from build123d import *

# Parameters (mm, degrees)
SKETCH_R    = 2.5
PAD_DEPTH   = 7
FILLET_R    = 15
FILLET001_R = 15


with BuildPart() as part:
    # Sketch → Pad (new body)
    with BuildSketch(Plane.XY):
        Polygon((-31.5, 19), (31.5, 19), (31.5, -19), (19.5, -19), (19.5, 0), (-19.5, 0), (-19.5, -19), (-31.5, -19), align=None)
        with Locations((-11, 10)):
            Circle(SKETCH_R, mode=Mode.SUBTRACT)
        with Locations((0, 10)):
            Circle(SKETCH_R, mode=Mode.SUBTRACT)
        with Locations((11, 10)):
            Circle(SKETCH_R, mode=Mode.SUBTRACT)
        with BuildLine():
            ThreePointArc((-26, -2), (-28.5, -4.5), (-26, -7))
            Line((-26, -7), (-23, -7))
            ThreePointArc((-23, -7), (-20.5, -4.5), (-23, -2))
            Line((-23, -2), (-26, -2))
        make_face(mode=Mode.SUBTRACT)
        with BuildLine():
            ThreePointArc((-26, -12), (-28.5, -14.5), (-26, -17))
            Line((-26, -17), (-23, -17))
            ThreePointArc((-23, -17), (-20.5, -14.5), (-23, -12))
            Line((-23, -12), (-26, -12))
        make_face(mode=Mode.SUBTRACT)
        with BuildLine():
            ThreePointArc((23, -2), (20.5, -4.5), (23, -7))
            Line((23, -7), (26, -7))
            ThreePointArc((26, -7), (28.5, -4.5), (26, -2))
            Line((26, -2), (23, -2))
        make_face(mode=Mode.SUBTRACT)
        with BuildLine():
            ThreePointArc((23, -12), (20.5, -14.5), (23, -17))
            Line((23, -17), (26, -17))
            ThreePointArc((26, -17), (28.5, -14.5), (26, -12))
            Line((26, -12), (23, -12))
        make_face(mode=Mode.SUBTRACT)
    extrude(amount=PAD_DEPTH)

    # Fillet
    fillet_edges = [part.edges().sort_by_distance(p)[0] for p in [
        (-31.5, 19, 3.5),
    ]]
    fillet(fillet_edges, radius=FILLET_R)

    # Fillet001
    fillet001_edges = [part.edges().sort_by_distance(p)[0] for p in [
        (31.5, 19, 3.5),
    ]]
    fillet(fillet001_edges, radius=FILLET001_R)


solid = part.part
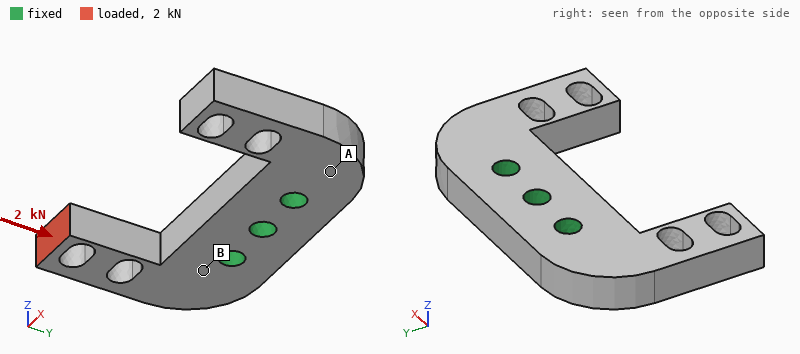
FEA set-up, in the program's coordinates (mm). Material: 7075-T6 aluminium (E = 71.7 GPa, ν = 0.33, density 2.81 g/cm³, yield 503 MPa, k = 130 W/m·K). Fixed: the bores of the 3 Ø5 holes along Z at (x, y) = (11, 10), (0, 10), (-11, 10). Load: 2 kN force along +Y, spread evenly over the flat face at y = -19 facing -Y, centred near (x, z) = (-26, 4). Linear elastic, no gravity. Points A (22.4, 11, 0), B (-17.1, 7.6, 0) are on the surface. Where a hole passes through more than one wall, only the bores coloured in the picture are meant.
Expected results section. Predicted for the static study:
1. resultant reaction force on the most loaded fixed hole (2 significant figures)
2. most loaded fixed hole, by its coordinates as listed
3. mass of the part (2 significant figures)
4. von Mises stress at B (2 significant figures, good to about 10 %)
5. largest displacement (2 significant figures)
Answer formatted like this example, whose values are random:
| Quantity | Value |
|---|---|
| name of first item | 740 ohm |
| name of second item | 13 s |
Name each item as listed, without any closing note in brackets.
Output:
| Quantity | Value |
|---|---|
| resultant reaction force on the most loaded fixed hole | 3.1 kN |
| most loaded fixed hole, by its coordinates as listed | (-11, 10) |
| mass of the part | 27 g |
| von Mises stress at B | 39 MPa |
| largest displacement | 68 µm |
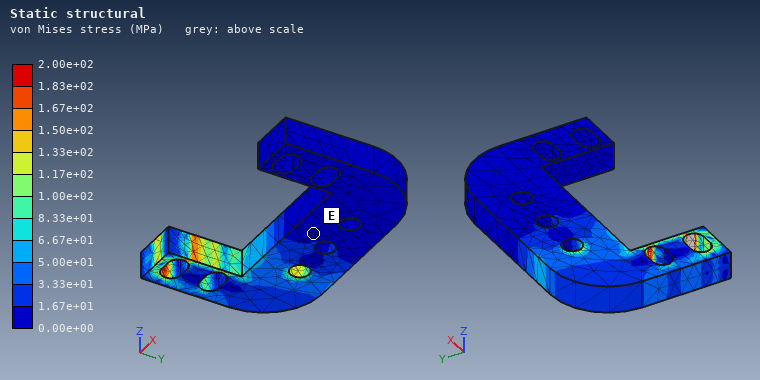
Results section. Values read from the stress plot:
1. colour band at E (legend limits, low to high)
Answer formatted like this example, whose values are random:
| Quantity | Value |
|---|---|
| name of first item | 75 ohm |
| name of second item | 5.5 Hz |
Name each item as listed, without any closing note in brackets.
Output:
| Quantity | Value |
|---|---|
| colour band at E | 0.00e+00 to 1.67e+01 MPa |
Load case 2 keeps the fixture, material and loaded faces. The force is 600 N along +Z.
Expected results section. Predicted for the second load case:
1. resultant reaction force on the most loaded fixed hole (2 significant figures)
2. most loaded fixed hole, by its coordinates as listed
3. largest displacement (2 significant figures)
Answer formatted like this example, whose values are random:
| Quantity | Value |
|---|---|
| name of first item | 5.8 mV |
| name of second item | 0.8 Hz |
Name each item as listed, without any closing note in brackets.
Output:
| Quantity | Value |
|---|---|
| resultant reaction force on the most loaded fixed hole | 760 N |
| most loaded fixed hole, by its coordinates as listed | (-11, 10) |
| largest displacement | 0.38 mm |
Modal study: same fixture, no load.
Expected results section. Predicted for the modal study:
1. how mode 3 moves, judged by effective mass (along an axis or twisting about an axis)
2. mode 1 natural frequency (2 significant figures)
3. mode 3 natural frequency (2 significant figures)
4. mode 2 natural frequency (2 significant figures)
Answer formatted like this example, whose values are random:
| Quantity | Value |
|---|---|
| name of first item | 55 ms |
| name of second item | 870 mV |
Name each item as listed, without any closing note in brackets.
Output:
| Quantity | Value |
|---|---|
| how mode 3 moves, judged by effective mass | along X |
| mode 1 natural frequency | 5800 Hz |
| mode 3 natural frequency | 9500 Hz |
| mode 2 natural frequency | 5800 Hz |
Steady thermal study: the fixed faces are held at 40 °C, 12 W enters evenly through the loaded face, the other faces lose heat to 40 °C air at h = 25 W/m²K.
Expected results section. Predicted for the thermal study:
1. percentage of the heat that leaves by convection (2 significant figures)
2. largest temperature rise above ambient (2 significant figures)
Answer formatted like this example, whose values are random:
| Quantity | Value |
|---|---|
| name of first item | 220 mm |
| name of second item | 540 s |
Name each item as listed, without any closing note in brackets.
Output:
| Quantity | Value |
|---|---|
| percentage of the heat that leaves by convection | 7.8 % |
| largest temperature rise above ambient | 60 K |
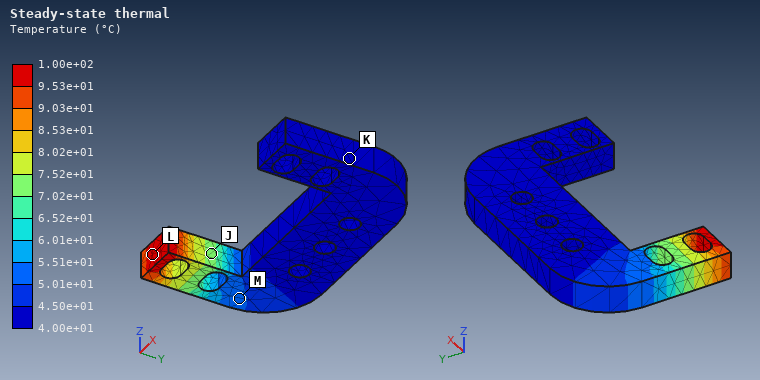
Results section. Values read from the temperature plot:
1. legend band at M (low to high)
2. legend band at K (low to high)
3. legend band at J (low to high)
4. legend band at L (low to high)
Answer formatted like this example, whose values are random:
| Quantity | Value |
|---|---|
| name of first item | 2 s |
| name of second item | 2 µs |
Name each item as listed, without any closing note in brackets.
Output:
| Quantity | Value |
|---|---|
| legend band at M | 5.01e+01 to 5.51e+01 °C |
| legend band at K | 4.00e+01 to 4.50e+01 °C |
| legend band at J | 7.02e+01 to 7.52e+01 °C |
| legend band at L | 9.53e+01 to 1.00e+02 °C |
